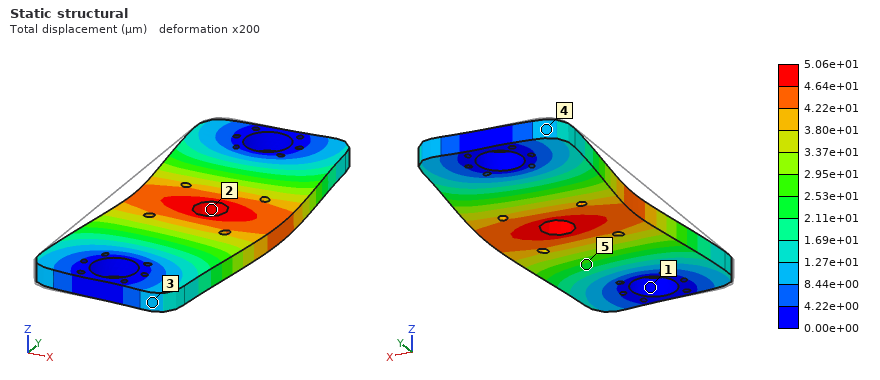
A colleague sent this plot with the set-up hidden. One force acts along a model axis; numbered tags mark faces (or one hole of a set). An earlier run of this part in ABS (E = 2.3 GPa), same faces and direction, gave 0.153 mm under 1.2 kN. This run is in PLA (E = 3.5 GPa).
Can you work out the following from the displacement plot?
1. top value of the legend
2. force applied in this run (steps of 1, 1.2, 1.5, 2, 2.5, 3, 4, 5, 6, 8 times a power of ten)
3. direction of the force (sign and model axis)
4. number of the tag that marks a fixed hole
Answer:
5.06e+01 µm
600 N
+X
1
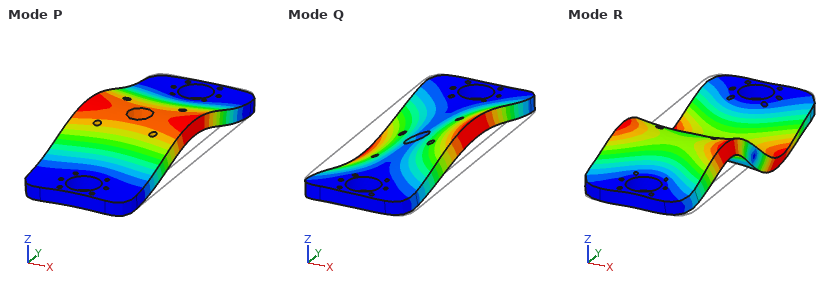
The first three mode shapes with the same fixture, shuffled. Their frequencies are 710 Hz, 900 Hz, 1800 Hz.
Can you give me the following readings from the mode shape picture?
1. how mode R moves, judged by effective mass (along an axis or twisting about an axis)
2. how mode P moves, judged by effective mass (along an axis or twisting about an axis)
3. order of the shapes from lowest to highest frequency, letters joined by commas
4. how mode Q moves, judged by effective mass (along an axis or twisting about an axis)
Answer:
twisting about X
along Z
P, Q, R
twisting about Y
